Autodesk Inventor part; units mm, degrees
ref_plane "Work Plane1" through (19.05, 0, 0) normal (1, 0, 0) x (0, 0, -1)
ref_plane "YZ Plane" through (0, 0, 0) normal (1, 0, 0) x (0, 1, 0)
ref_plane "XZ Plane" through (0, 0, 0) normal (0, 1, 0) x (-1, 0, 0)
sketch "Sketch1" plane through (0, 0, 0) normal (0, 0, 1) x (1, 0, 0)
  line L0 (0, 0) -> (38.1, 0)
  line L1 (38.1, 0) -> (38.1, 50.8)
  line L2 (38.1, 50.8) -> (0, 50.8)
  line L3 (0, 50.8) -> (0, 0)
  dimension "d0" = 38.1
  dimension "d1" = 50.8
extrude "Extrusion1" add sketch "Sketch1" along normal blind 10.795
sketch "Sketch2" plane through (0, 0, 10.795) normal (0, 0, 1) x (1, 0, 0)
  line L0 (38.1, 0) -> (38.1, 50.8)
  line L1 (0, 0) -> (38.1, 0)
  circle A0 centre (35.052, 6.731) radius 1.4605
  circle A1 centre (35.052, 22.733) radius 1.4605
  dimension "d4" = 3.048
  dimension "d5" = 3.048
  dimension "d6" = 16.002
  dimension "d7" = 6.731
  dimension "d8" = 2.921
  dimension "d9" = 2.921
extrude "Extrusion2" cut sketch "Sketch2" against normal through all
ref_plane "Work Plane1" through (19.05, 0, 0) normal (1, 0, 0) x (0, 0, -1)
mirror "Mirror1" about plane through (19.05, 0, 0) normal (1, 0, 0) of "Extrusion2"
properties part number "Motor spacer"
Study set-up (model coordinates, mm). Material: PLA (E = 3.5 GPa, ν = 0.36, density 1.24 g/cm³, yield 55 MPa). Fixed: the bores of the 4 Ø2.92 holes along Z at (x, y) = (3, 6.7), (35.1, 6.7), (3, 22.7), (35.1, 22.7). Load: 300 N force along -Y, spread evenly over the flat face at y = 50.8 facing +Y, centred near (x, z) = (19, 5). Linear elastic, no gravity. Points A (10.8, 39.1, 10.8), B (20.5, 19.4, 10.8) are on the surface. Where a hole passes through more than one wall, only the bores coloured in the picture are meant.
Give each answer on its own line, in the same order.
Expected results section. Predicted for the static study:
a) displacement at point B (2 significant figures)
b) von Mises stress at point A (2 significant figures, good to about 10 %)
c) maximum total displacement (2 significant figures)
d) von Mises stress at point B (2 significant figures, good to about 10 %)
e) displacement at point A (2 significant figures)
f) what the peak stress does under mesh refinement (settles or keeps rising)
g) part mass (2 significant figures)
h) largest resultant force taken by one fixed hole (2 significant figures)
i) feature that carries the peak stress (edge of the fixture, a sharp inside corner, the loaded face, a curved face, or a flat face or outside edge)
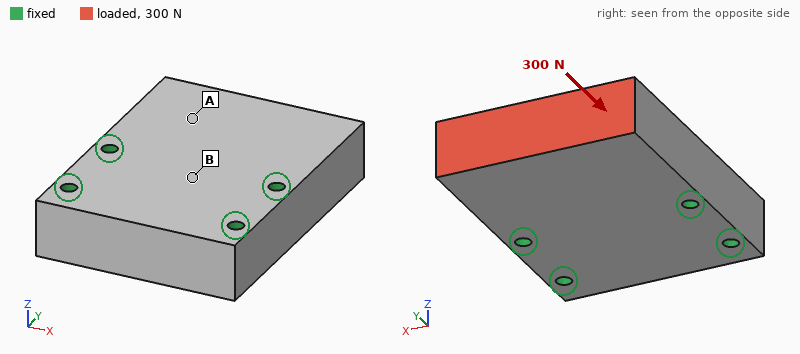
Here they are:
2.4 µm
0.69 MPa
7.1 µm
0.30 MPa
4.7 µm
keeps rising
26 g
120 N
edge of the fixture
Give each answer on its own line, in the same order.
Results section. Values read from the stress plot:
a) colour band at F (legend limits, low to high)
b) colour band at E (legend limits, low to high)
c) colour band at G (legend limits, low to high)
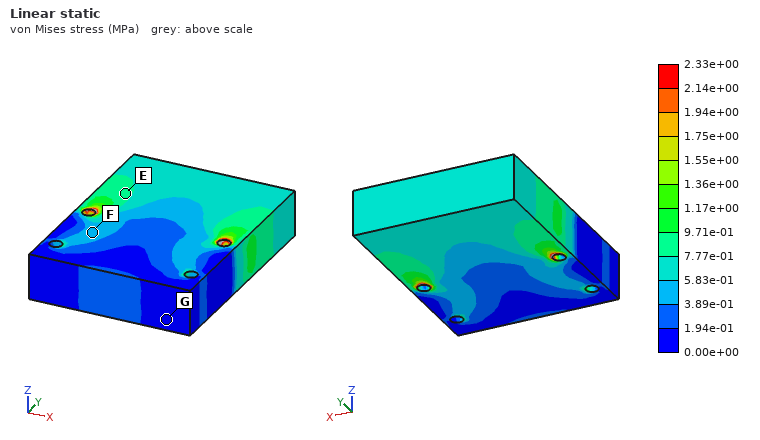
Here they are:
3.89e-01 to 5.83e-01 MPa
7.77e-01 to 9.71e-01 MPa
0.00e+00 to 1.94e-01 MPa
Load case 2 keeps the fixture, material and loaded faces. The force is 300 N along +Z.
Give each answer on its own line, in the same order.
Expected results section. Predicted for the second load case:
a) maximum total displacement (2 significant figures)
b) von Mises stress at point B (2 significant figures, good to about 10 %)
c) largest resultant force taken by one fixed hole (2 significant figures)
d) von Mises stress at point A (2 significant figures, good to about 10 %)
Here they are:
0.24 mm
4.7 MPa
230 N
4.8 MPa
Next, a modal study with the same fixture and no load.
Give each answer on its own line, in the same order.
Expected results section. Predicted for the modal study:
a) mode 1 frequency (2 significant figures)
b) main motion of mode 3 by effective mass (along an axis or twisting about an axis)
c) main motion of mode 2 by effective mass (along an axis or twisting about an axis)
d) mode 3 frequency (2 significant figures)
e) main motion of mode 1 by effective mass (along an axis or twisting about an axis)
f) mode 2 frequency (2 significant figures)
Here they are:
2800 Hz
along X
twisting about Y
6700 Hz
along Z
5500 Hz
